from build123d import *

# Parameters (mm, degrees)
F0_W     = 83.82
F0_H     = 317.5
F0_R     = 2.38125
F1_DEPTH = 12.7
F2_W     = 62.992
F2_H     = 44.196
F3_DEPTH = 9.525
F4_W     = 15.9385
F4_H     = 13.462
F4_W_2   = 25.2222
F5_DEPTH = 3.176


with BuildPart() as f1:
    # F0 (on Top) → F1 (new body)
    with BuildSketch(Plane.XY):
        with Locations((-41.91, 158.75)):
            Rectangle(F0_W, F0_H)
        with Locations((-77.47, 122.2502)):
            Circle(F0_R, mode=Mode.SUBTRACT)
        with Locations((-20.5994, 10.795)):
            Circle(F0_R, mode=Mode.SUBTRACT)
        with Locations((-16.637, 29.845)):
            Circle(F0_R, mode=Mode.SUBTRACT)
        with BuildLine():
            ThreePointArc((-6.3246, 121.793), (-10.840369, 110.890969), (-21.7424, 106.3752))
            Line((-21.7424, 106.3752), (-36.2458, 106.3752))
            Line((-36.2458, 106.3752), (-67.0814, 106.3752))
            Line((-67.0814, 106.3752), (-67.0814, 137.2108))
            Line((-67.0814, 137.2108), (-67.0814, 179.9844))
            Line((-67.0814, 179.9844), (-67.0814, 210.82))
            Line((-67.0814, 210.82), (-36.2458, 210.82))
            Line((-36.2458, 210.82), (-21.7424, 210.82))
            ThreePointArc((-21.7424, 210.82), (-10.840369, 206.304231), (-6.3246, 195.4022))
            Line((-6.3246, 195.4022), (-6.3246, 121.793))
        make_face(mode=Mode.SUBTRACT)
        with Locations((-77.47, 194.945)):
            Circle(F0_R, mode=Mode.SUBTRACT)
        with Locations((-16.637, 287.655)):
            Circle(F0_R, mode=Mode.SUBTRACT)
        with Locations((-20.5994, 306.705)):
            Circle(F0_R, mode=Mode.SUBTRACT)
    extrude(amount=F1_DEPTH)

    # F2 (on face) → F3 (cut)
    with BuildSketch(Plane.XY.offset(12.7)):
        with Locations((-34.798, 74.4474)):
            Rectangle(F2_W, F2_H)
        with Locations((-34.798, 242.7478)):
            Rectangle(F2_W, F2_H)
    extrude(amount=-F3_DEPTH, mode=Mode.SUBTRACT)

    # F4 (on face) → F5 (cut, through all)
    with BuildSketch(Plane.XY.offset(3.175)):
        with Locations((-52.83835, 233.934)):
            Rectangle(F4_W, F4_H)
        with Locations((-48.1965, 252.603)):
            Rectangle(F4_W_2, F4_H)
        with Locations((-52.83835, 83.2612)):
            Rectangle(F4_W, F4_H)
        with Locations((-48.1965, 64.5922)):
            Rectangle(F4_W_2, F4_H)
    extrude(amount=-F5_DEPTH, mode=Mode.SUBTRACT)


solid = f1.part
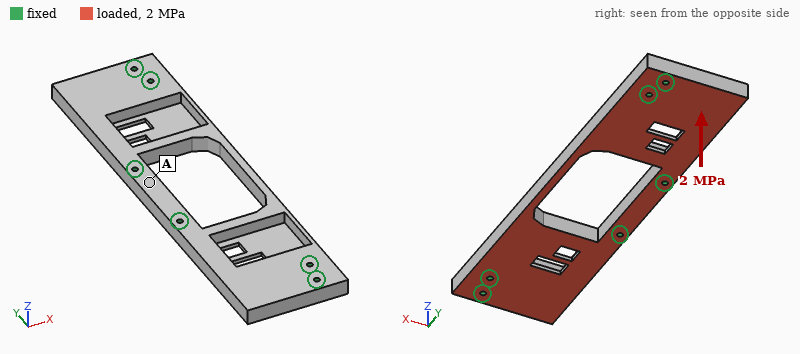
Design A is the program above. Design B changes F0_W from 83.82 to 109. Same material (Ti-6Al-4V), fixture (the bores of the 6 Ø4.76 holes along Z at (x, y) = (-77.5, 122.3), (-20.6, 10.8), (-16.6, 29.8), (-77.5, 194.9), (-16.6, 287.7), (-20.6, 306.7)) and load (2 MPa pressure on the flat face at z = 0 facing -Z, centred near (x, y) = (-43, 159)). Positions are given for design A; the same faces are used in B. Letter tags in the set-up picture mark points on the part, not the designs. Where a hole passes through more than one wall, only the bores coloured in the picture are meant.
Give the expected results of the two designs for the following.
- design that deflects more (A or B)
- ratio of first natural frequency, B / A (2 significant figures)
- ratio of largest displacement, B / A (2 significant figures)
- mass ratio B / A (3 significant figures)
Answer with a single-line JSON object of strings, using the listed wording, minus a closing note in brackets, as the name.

{"design that deflects more": "B", "ratio of first natural frequency, B / A": "0.82", "ratio of largest displacement, B / A": "1.2", "mass ratio B / A": "1.51"}
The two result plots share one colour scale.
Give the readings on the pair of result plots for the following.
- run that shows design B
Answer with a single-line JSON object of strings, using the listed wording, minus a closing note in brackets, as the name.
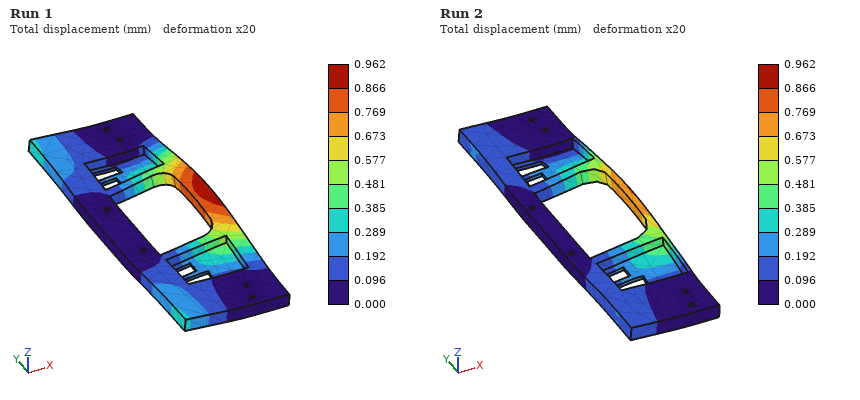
{"run that shows design B": "Run 1"}
